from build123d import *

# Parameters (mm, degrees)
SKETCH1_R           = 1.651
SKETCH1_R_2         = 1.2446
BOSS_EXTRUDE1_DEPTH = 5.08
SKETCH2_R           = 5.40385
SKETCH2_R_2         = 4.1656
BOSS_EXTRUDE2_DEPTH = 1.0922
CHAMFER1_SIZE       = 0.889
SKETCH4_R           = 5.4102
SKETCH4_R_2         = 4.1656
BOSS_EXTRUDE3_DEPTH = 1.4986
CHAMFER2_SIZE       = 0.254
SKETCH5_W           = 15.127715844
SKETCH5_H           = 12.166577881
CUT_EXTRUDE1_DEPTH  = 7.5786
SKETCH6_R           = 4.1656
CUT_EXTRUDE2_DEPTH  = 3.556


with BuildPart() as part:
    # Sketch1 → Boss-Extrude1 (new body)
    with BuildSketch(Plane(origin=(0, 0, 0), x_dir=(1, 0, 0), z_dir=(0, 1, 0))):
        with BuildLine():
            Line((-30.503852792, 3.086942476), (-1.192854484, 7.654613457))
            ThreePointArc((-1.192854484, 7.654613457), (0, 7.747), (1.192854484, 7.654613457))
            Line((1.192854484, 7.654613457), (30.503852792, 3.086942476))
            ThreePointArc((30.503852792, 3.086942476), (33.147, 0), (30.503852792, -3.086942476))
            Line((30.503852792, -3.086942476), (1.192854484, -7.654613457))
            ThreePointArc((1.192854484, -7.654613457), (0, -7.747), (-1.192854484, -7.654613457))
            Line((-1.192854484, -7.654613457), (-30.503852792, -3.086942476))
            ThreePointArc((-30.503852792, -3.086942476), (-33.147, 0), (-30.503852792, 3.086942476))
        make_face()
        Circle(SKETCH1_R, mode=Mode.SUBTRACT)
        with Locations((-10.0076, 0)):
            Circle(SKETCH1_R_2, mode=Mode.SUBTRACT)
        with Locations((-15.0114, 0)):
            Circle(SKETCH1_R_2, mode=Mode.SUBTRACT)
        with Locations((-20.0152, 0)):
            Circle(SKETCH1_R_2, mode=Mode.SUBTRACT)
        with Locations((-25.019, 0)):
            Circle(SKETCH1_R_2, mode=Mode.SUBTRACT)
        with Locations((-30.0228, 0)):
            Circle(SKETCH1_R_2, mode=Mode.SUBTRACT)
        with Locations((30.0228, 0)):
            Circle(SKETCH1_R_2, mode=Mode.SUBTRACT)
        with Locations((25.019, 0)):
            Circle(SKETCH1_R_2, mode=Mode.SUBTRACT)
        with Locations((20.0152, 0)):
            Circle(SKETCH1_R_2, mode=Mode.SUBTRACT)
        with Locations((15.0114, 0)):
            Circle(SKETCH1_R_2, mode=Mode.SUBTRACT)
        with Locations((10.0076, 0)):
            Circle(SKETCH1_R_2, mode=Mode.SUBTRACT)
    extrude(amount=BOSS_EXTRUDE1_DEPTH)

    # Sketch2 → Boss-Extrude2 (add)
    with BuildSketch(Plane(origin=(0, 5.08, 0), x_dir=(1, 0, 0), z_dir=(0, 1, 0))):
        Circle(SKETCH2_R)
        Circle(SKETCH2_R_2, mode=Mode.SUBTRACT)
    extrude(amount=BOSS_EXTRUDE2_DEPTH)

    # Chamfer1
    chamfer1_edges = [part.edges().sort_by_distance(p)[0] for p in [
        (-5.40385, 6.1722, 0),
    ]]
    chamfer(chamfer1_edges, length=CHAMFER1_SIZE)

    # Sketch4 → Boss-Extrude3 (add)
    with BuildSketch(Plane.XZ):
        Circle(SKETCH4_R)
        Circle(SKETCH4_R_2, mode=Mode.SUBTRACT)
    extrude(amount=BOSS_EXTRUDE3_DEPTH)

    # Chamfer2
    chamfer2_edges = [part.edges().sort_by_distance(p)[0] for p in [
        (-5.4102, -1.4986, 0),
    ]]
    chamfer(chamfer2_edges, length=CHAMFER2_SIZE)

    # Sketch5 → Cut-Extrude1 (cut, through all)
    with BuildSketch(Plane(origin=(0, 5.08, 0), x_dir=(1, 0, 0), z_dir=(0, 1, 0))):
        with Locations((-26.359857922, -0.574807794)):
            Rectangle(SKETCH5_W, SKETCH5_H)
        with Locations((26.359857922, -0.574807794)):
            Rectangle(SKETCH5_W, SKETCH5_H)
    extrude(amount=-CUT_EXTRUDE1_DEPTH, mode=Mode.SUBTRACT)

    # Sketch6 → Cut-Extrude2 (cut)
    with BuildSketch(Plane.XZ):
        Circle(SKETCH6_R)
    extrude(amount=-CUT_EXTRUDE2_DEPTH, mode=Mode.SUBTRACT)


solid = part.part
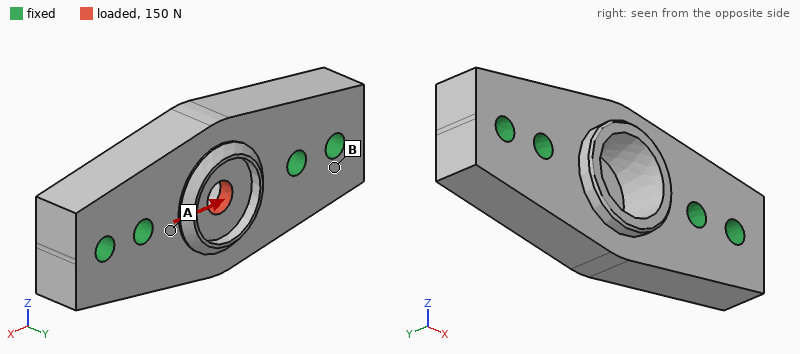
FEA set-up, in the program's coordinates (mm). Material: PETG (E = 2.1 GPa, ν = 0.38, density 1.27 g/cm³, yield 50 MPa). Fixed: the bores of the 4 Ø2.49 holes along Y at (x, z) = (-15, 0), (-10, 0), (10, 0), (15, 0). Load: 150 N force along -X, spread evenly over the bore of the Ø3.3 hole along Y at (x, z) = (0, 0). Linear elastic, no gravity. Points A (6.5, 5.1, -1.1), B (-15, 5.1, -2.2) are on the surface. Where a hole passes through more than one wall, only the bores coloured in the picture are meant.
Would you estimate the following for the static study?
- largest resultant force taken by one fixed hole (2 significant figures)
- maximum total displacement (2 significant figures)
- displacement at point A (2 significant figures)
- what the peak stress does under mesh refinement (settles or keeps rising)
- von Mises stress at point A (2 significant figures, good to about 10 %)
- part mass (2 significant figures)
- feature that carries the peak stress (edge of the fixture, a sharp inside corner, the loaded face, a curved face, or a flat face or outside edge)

59 N
22 µm
5.1 µm
keeps rising
4.4 MPa
2.8 g
a sharp inside corner
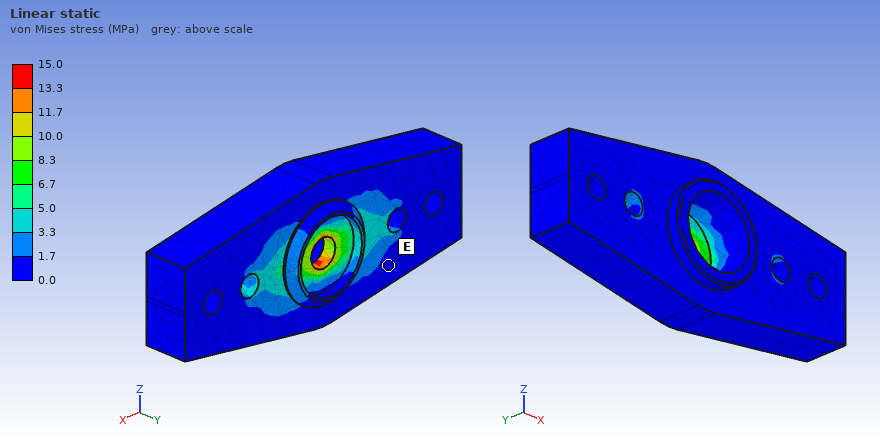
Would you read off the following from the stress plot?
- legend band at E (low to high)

0.0 to 1.7 MPa
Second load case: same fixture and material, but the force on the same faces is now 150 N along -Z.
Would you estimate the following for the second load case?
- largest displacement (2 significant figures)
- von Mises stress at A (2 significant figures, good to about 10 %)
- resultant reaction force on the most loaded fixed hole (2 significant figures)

39 µm
3.6 MPa
90 N
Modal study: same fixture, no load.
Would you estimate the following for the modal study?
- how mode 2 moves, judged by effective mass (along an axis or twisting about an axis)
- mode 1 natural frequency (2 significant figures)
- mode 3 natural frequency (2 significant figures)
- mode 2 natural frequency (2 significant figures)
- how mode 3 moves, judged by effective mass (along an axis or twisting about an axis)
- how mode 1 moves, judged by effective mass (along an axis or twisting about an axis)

along Y
10 kHz
16 kHz
11 kHz
along Z
twisting about X
